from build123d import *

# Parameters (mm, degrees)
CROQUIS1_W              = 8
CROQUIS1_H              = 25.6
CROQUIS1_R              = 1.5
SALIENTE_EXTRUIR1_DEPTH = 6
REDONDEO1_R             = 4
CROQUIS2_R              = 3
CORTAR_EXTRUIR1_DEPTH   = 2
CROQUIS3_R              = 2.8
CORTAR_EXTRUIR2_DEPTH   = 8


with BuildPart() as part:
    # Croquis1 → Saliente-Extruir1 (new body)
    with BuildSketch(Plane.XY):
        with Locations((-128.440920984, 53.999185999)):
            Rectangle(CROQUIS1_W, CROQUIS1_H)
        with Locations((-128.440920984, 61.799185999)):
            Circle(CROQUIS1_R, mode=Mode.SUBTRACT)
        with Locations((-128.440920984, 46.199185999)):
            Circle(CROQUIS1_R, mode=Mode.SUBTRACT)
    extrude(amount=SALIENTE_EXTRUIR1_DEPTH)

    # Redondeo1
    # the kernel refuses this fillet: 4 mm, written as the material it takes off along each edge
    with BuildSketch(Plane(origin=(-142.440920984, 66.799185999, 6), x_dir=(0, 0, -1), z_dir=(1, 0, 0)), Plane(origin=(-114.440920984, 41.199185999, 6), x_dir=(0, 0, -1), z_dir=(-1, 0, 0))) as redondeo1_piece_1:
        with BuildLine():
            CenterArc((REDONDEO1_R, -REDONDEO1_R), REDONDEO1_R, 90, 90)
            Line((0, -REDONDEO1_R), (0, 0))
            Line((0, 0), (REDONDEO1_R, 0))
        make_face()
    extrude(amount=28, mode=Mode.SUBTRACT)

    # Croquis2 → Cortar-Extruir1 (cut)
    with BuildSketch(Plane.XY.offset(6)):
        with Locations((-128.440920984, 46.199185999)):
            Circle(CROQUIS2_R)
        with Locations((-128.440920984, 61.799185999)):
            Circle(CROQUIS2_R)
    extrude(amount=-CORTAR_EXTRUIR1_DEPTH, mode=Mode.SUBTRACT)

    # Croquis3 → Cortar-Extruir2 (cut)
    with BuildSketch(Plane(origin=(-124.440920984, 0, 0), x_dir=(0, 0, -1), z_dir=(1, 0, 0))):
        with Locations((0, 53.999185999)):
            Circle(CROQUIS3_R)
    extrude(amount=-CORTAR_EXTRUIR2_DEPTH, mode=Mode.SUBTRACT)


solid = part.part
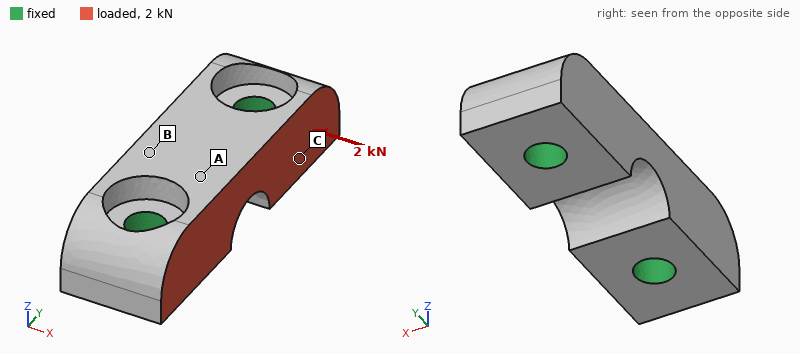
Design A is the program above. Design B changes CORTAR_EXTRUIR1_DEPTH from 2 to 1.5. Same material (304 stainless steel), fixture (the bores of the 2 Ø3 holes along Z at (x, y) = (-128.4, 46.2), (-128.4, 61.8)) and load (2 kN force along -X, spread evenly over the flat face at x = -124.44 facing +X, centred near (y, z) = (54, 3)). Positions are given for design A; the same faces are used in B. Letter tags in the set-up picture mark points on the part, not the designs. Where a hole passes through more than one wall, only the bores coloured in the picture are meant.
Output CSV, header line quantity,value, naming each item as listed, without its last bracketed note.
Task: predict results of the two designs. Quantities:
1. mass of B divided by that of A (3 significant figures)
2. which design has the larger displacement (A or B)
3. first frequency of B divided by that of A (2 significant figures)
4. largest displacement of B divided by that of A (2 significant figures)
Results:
quantity,value
mass of B divided by that of A,1.02
which design has the larger displacement,A
first frequency of B divided by that of A,1.1
largest displacement of B divided by that of A,0.78
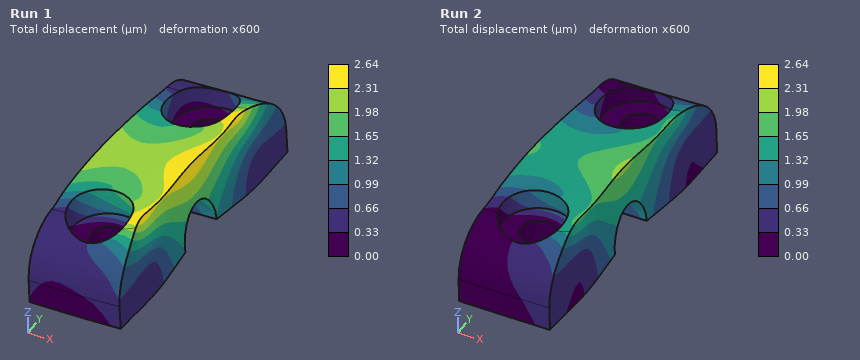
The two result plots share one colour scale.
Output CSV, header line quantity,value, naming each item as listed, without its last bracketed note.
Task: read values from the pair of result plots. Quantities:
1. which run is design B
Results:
quantity,value
which run is design B,Run 2
